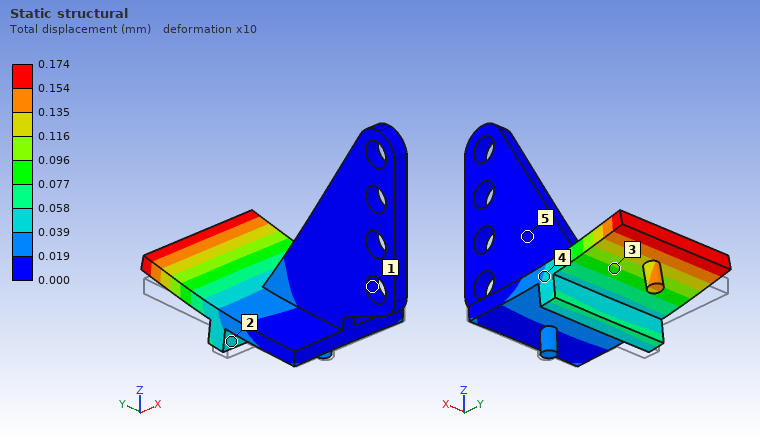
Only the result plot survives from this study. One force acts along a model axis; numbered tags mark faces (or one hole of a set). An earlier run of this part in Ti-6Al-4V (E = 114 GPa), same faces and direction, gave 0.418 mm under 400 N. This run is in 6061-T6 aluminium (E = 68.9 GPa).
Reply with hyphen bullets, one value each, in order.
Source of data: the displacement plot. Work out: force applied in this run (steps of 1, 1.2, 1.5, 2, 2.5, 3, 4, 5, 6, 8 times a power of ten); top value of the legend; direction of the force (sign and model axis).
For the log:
- 100 N
- 0.174 mm
- +Z
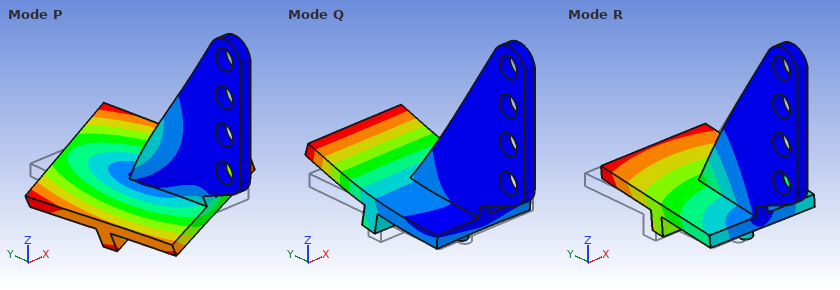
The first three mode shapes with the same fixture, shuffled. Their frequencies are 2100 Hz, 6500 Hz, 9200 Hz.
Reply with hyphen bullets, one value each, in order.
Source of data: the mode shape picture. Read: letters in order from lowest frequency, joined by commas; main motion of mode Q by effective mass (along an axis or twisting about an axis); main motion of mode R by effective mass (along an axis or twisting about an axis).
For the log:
- R, P, Q
- along Z
- along X
